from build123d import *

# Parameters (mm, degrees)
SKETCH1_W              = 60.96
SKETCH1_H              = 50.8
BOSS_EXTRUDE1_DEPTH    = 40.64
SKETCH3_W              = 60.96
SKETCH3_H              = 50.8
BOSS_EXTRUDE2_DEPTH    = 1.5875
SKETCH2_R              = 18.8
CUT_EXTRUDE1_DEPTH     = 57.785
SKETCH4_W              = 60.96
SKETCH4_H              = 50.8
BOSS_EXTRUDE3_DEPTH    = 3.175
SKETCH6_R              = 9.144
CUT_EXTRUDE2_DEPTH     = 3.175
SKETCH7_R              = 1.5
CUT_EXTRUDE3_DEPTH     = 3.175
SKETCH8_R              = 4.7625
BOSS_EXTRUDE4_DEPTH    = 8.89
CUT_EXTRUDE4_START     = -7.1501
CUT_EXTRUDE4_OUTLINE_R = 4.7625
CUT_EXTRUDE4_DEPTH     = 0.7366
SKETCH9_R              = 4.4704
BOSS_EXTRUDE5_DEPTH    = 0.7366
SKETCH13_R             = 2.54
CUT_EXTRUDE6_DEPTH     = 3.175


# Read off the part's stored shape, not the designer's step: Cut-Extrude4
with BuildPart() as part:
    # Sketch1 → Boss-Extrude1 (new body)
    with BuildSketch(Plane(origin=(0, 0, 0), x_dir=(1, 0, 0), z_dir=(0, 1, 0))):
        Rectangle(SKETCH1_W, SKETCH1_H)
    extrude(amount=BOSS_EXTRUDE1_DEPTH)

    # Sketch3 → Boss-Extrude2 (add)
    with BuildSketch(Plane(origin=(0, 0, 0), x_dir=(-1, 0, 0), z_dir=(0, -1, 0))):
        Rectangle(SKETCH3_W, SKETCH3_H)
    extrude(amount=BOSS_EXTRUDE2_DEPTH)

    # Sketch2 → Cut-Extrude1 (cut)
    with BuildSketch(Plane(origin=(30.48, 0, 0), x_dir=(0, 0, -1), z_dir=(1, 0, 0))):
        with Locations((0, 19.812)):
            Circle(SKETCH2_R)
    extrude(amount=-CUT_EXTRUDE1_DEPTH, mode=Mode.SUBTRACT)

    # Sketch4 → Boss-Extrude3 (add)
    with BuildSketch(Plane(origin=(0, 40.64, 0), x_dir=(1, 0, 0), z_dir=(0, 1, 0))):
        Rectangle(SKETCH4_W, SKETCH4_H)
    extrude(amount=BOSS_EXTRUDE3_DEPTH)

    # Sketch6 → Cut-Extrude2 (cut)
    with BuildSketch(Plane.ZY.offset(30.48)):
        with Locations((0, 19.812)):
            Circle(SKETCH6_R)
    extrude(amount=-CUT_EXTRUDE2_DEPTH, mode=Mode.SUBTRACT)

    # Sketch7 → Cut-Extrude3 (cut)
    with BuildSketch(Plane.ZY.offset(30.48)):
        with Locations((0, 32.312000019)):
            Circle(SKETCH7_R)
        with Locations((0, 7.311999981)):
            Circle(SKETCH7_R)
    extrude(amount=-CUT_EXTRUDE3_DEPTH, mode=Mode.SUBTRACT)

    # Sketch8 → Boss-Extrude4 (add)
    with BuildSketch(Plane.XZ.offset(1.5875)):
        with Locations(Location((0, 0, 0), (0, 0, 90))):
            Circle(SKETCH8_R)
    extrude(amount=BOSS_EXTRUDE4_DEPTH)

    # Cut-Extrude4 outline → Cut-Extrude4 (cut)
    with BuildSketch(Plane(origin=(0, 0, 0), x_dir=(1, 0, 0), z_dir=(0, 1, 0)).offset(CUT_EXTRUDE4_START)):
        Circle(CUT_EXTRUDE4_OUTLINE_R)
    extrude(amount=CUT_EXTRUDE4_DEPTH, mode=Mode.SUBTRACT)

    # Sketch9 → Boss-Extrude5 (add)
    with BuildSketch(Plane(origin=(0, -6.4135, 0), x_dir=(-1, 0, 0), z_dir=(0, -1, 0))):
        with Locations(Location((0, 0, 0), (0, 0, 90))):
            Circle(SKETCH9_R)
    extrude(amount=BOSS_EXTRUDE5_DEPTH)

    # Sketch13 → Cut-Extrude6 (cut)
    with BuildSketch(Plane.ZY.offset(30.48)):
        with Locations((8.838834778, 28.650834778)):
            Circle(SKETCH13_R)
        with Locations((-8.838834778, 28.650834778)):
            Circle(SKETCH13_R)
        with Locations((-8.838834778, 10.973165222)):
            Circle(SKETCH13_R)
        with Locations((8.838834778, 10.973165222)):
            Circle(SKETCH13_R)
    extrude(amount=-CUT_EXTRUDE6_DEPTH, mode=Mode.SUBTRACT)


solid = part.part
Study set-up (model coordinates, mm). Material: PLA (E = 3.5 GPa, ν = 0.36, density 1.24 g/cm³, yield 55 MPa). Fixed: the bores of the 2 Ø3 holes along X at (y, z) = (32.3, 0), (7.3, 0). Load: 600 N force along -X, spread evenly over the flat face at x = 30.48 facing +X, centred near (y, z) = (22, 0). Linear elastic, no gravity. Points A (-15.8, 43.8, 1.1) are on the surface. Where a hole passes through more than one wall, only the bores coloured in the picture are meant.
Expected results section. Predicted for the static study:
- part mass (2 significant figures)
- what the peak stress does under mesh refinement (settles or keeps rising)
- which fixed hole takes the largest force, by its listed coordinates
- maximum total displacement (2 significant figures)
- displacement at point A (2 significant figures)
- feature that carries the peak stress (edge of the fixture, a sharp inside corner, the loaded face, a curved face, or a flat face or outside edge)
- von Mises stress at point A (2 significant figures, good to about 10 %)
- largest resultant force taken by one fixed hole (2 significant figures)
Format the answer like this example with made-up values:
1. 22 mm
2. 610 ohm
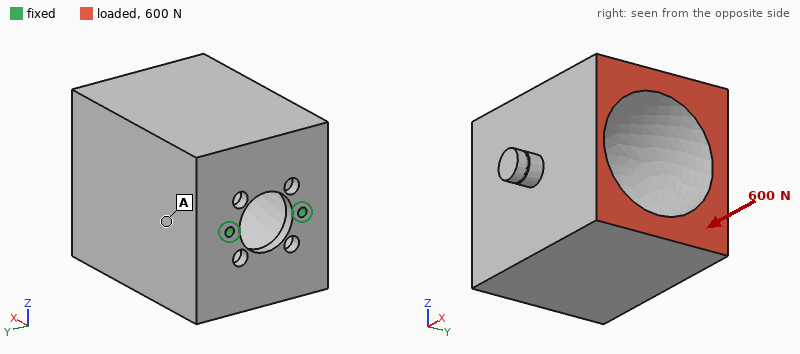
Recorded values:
1. 94 g
2. keeps rising
3. (32.3, 0)
4. 0.16 mm
5. 0.14 mm
6. edge of the fixture
7. 2.4 MPa
8. 350 N
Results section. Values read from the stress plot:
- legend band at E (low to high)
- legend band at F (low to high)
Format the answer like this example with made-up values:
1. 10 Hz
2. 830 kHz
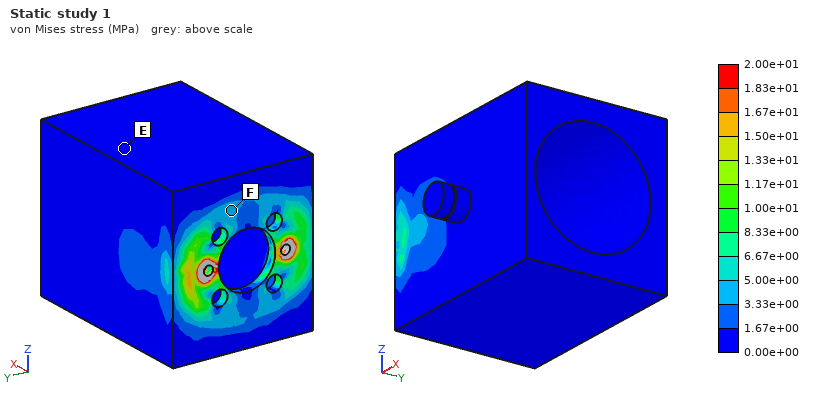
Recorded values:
1. 0.00e+00 to 1.67e+00 MPa
2. 3.33e+00 to 5.00e+00 MPa
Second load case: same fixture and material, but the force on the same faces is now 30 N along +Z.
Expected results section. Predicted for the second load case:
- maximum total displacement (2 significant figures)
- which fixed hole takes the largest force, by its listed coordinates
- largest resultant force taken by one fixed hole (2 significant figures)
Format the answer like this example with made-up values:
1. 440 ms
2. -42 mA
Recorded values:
1. 1.0 mm
2. (32.3, 0)
3. 17 N
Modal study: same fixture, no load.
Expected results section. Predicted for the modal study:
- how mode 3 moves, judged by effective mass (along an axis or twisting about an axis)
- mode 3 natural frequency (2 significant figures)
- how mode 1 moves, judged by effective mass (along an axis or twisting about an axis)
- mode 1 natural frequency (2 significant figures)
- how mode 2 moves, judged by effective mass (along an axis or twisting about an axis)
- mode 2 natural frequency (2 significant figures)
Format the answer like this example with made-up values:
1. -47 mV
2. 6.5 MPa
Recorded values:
1. twisting about X
2. 1100 Hz
3. along Z
4. 140 Hz
5. along Y
6. 450 Hz
